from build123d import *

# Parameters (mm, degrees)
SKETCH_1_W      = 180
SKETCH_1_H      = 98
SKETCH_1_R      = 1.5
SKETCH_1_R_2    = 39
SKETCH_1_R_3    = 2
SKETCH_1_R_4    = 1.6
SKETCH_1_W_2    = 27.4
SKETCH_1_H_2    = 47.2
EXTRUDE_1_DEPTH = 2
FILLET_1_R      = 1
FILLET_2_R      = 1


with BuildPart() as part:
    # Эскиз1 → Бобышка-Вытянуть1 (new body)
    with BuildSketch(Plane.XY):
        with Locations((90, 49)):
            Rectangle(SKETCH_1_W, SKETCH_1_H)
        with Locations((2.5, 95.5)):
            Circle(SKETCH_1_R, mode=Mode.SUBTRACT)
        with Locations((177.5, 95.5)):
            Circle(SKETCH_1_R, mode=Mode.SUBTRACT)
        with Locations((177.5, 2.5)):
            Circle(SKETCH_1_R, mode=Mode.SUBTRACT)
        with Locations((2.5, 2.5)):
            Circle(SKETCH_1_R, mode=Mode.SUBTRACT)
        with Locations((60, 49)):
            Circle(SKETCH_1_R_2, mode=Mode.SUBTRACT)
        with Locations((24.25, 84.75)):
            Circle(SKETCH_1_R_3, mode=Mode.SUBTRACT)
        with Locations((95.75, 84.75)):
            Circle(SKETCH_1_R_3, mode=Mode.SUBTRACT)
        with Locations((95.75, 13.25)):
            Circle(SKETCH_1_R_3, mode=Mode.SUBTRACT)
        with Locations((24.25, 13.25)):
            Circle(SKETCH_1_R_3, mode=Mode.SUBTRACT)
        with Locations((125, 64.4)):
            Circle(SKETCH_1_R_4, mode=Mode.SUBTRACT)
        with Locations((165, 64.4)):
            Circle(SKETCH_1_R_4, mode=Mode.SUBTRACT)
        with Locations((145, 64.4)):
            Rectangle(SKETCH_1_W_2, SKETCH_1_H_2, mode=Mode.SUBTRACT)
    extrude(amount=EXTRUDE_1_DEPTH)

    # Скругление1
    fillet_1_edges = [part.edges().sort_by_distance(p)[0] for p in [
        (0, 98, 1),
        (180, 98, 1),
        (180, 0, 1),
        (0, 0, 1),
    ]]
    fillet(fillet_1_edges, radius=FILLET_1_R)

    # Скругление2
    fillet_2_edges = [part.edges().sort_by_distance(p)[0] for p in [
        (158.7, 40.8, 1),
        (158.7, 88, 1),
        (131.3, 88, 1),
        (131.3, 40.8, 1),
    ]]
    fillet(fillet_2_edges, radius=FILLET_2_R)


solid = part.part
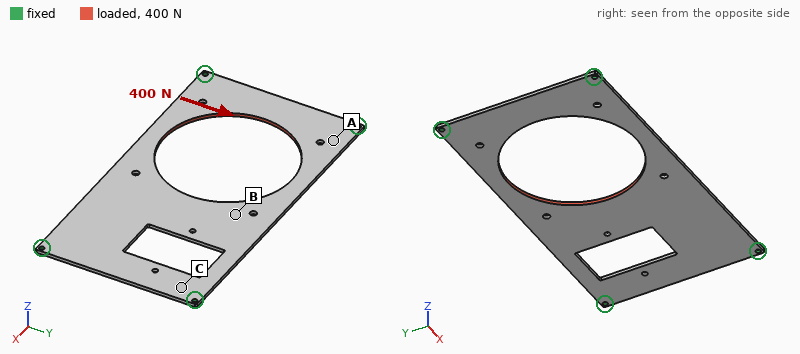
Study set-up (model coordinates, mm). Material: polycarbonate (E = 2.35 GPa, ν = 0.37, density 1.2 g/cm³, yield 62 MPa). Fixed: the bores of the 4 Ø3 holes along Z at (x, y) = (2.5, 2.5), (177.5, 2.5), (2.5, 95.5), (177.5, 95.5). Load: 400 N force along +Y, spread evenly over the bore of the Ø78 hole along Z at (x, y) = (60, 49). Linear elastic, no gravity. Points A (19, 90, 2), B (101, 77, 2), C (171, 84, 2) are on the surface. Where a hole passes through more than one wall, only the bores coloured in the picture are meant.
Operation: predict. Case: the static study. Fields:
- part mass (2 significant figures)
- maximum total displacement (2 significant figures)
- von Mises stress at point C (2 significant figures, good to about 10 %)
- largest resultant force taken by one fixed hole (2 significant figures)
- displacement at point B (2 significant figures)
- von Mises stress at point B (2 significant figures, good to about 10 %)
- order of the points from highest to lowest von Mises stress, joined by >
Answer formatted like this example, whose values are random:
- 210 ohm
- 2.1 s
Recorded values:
- 28 g
- 0.56 mm
- 3.6 MPa
- 140 N
- 0.41 mm
- 2.1 MPa
- C > B > A
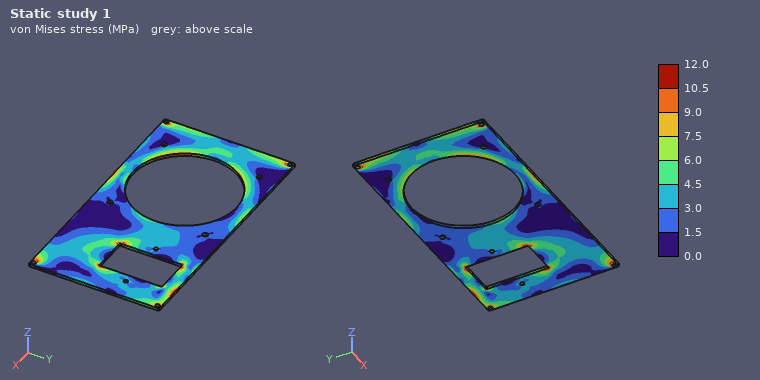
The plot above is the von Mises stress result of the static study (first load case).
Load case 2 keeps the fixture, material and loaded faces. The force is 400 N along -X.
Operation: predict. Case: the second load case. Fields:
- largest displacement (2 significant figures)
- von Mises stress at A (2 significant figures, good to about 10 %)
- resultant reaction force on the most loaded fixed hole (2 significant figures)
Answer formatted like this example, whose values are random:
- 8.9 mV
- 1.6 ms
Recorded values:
- 0.19 mm
- 2.8 MPa
- 140 N
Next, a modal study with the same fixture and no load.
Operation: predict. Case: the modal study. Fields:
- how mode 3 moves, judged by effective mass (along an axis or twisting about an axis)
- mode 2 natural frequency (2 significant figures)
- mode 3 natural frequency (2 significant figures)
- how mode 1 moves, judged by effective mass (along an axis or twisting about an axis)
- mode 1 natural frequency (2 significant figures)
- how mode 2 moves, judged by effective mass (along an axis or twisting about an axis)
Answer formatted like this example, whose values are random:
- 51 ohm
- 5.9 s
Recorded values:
- twisting about Y
- 120 Hz
- 210 Hz
- along Z
- 74 Hz
- twisting about X
